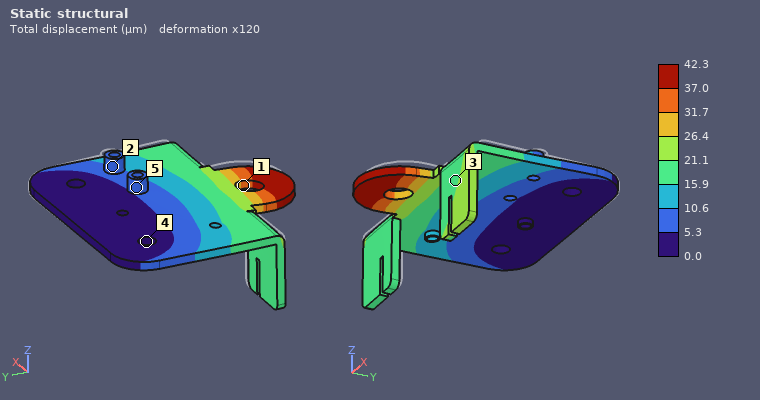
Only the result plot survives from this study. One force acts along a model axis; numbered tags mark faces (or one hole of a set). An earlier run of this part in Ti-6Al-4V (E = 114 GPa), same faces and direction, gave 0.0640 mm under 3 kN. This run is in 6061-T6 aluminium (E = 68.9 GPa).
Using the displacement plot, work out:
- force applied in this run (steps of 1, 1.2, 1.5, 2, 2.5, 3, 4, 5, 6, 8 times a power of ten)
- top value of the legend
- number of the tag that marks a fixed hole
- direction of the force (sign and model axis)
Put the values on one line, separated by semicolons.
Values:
1.2 kN; 42.3 µm; 4; -X
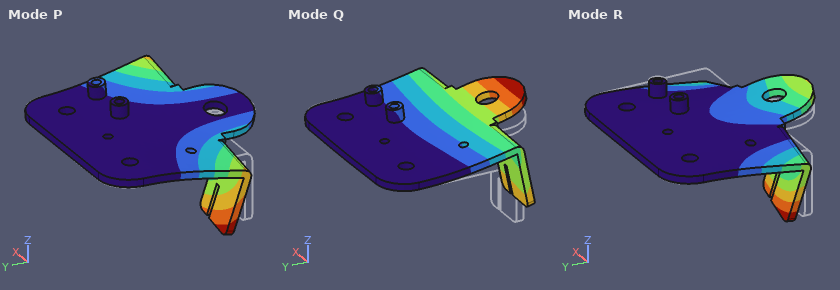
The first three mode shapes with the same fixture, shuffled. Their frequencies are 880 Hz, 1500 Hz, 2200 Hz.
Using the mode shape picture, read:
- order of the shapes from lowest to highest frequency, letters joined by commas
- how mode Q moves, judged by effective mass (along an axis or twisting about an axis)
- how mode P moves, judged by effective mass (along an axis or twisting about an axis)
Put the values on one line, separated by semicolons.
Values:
Q, P, R; along Z; twisting about Y
